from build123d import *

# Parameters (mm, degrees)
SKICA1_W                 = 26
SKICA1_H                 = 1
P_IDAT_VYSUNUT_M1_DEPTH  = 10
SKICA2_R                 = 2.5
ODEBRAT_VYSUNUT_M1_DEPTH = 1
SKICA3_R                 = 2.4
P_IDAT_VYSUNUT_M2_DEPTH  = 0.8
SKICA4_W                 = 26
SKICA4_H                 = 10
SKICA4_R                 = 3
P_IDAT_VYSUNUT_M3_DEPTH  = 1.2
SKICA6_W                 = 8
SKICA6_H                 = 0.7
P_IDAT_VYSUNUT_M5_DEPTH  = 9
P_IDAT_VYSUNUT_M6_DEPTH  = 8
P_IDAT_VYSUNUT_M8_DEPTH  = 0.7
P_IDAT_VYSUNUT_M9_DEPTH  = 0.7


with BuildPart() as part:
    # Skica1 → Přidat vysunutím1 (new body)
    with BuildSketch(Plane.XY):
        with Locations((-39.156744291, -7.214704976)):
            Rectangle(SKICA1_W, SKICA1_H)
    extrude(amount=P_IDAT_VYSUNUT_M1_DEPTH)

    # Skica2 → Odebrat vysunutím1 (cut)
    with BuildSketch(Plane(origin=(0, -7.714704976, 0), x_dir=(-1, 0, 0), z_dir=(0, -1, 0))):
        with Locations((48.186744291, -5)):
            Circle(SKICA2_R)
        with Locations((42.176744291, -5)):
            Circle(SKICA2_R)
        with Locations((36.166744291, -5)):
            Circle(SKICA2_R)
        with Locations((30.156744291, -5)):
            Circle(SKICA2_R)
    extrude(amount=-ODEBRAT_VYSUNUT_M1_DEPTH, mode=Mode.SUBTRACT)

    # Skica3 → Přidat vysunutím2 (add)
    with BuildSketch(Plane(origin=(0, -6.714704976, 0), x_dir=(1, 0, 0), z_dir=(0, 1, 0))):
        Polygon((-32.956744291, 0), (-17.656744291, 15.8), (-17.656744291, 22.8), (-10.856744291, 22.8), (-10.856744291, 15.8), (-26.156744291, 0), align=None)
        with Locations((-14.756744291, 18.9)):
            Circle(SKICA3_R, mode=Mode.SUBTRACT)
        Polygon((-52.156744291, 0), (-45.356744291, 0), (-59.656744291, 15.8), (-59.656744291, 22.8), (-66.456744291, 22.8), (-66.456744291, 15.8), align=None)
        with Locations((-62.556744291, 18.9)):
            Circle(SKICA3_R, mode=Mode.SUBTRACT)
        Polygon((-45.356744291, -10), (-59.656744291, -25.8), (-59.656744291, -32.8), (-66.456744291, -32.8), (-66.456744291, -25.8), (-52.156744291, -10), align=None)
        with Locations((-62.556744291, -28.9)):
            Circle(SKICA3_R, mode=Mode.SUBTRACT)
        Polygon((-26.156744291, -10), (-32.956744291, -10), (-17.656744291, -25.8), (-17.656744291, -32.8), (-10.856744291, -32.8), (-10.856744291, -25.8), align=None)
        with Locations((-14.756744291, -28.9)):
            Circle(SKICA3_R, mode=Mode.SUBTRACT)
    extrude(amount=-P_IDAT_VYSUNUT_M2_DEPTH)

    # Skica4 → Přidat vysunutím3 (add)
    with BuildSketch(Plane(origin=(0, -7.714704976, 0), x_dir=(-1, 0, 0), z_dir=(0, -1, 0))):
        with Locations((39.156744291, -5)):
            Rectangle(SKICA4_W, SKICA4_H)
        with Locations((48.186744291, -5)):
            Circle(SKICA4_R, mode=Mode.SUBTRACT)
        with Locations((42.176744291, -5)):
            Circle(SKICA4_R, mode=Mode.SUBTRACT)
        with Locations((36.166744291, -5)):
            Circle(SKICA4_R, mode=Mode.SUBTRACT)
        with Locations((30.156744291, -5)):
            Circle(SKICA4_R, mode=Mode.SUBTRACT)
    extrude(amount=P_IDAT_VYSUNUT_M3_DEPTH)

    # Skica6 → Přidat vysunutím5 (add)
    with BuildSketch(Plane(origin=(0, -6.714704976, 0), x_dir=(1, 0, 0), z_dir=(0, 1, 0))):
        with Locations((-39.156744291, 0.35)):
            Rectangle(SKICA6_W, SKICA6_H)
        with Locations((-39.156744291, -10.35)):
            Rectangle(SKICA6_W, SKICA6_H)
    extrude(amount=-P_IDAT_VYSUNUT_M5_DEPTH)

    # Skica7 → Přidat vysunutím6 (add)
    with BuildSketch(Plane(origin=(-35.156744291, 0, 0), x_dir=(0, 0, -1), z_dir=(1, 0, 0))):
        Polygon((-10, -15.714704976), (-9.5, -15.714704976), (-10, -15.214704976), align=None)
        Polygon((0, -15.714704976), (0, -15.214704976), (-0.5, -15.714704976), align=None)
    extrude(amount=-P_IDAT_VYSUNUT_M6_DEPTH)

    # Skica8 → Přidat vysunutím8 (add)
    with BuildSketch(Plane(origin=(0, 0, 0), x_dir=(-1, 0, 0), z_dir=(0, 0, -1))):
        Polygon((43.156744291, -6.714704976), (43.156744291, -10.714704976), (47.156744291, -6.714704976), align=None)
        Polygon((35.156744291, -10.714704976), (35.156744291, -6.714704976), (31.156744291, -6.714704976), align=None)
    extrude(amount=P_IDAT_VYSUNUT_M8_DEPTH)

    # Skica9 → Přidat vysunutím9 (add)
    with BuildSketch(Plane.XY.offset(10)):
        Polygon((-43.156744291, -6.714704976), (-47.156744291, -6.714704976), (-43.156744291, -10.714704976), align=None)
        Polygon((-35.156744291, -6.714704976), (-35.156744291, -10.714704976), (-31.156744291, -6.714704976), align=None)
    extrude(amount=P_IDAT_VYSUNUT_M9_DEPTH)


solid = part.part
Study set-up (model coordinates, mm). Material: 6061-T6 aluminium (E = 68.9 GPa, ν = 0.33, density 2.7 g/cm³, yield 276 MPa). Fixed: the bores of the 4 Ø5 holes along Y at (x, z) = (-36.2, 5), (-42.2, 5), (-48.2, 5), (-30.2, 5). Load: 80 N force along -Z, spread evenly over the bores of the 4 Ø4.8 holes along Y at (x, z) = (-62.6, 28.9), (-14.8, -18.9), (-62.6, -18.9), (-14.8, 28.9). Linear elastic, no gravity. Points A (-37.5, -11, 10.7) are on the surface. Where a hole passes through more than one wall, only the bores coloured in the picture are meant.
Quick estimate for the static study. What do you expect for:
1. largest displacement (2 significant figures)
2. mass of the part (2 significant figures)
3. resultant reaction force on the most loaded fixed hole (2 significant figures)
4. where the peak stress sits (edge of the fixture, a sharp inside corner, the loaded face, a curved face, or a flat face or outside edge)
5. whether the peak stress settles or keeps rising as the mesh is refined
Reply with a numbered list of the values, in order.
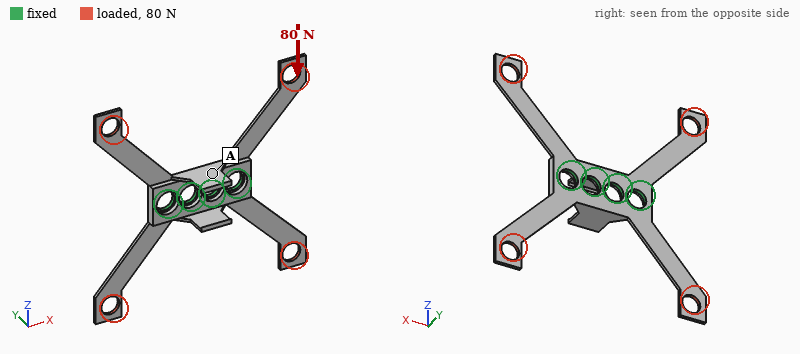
1. 0.14 mm
2. 2.5 g
3. 82 N
4. a sharp inside corner
5. keeps rising
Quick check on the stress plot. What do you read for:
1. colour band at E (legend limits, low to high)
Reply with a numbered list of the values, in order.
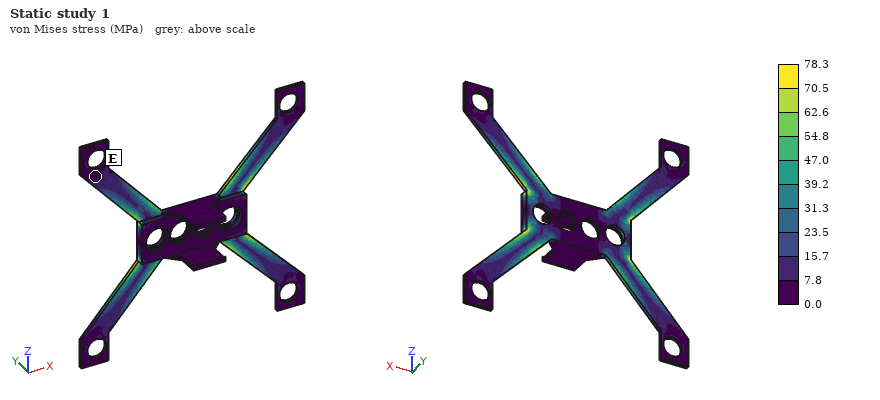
1. 0.0 to 7.8 MPa
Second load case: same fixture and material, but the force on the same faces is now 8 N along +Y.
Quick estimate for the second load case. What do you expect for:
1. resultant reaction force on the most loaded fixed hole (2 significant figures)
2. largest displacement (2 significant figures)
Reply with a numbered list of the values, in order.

1. 15 N
2. 0.81 mm
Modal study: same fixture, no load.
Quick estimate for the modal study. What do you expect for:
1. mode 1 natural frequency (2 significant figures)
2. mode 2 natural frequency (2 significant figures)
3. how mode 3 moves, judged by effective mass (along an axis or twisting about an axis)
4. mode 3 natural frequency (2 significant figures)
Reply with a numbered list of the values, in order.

1. 860 Hz
2. 870 Hz
3. twisting about X
4. 910 Hz
